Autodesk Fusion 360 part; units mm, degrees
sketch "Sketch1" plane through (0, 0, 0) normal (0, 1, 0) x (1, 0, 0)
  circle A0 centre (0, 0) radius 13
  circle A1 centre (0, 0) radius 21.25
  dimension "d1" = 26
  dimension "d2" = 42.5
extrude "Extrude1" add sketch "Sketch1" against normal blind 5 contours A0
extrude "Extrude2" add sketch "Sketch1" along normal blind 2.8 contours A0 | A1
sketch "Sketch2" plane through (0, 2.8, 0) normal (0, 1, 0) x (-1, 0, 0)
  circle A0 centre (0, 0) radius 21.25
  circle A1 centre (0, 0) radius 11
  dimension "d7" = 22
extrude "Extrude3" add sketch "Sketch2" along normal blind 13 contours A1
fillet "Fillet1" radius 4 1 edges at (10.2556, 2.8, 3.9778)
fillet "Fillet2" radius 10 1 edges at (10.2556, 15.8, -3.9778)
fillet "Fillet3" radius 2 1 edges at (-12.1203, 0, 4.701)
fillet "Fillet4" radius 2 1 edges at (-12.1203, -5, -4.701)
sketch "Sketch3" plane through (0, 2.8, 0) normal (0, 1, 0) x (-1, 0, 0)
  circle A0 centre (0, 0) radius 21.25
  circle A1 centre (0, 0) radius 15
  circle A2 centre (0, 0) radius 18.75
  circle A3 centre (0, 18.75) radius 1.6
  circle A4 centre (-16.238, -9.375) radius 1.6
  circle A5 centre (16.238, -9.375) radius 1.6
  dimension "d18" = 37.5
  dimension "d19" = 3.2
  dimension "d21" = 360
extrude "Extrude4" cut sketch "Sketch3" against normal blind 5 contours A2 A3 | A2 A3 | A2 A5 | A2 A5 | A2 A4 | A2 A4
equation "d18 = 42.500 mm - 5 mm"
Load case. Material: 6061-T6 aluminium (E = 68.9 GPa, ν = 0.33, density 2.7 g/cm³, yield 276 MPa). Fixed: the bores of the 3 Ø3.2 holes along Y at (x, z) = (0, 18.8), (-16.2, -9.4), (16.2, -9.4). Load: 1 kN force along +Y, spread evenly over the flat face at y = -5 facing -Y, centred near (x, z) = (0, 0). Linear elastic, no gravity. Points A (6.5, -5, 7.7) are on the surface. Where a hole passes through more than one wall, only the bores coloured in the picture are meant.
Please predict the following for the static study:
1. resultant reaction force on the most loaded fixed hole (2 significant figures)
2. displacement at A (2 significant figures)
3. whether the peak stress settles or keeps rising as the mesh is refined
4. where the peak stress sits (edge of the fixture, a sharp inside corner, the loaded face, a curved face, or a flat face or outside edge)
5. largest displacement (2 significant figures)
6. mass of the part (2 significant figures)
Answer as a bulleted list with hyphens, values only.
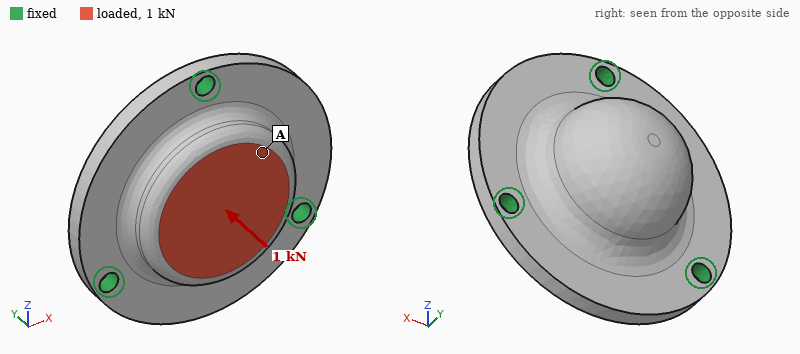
- 340 N
- 6.8 µm
- keeps rising
- edge of the fixture
- 7.4 µm
- 29 g
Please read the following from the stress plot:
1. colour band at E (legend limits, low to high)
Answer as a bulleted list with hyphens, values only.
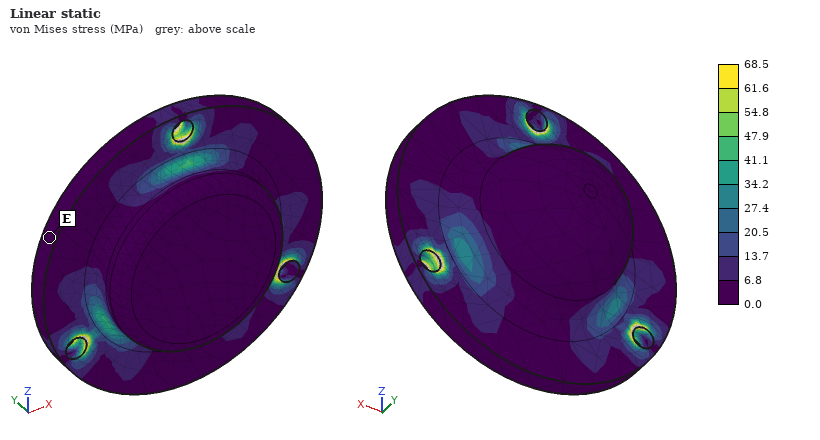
- 0.0 to 6.8 MPa
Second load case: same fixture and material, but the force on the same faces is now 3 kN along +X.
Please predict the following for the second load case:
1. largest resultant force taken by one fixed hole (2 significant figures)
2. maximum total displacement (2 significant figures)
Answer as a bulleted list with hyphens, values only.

- 1.3 kN
- 21 µm
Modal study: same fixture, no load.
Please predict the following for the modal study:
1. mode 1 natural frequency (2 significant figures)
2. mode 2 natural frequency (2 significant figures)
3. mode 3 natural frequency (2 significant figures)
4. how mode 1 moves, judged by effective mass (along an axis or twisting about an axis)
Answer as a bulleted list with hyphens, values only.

- 12 kHz
- 15 kHz
- 15 kHz
- along Y
